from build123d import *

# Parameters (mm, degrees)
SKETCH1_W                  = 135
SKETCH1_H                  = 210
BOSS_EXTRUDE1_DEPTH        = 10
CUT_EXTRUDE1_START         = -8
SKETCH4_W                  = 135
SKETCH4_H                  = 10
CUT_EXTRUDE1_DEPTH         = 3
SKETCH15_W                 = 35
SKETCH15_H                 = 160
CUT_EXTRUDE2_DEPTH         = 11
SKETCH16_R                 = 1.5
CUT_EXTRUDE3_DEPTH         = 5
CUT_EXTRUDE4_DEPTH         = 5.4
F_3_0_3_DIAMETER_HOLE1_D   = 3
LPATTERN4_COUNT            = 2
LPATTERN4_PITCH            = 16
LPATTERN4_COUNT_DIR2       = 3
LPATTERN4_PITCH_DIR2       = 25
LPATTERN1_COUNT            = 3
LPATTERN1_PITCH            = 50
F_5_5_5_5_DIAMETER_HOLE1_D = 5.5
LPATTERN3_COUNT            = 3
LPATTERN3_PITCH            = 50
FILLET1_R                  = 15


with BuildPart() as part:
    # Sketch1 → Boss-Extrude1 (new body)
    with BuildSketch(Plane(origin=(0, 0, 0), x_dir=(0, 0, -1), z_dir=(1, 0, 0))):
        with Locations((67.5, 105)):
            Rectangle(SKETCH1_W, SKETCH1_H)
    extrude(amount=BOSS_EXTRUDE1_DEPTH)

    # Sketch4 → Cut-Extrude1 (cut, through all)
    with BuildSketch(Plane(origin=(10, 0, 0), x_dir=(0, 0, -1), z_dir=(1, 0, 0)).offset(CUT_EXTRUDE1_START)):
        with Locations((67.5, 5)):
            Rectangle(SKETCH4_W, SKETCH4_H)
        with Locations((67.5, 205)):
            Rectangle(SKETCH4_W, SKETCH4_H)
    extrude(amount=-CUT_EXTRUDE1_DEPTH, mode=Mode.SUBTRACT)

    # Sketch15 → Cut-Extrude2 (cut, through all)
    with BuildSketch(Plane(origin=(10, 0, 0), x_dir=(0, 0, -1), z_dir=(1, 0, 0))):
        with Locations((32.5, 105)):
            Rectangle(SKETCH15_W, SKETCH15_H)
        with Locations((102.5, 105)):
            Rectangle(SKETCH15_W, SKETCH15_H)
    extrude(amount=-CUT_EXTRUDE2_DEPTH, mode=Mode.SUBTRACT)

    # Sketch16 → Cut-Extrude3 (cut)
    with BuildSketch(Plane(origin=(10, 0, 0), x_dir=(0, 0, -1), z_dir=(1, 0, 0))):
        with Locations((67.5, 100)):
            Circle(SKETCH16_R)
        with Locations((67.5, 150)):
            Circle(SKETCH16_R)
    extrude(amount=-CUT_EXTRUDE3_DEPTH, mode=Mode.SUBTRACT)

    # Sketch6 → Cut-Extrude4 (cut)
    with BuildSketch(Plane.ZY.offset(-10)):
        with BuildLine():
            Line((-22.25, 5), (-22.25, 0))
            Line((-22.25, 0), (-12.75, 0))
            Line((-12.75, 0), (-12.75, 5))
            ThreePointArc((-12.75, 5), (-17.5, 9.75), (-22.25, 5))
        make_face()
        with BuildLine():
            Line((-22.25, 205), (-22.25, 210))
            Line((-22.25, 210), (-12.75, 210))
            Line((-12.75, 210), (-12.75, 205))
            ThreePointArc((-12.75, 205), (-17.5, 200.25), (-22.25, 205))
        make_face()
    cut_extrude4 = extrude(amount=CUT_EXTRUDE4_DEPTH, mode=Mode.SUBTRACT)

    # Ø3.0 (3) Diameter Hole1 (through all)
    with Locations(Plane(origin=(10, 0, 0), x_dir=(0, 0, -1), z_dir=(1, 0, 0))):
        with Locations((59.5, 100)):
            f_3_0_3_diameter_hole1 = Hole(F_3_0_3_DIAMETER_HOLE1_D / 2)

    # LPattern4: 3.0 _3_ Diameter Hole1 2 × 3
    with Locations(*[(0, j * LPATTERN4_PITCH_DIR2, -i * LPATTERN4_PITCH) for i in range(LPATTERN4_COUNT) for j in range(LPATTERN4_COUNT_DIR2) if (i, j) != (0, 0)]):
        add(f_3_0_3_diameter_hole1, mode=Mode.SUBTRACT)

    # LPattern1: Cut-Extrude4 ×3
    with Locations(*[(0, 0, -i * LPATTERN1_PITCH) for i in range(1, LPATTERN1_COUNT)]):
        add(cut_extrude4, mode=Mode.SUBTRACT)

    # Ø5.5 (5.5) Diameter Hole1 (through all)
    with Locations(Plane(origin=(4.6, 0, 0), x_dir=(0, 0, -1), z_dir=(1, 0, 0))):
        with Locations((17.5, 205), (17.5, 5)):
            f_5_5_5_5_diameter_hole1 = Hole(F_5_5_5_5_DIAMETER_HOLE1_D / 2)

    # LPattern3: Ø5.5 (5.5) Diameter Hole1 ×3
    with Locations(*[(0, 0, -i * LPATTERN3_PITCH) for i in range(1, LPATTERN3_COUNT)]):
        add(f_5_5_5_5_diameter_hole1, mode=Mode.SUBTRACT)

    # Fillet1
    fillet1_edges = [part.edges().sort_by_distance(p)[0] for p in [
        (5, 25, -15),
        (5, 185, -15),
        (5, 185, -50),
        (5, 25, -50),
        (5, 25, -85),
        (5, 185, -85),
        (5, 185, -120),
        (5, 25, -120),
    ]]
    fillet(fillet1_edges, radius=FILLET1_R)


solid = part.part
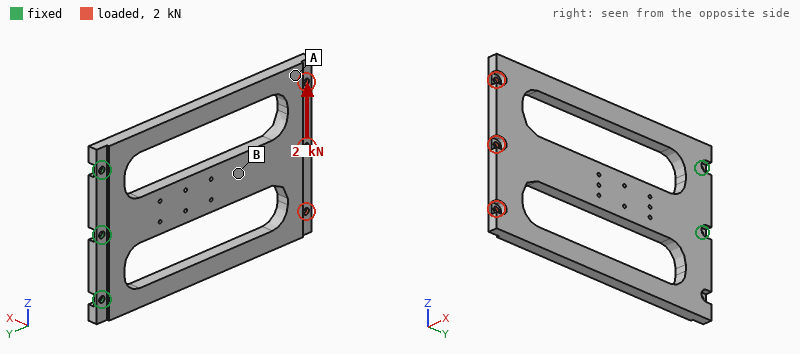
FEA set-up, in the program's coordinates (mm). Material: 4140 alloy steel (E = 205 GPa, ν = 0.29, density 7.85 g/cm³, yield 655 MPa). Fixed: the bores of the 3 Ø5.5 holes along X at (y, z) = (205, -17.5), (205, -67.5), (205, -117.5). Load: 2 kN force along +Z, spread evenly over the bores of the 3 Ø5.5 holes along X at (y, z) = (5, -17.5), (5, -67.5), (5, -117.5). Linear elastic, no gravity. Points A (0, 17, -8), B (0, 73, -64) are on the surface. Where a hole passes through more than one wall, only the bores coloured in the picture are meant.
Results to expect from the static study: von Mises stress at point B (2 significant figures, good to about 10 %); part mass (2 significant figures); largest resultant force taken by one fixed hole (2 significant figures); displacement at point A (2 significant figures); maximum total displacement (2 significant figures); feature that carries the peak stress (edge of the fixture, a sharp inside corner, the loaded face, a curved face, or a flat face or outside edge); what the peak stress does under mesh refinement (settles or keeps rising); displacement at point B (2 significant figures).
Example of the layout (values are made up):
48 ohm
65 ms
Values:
16 MPa
1.3 kg
4.0 kN
0.16 mm
0.16 mm
edge of the fixture
keeps rising
0.11 mm
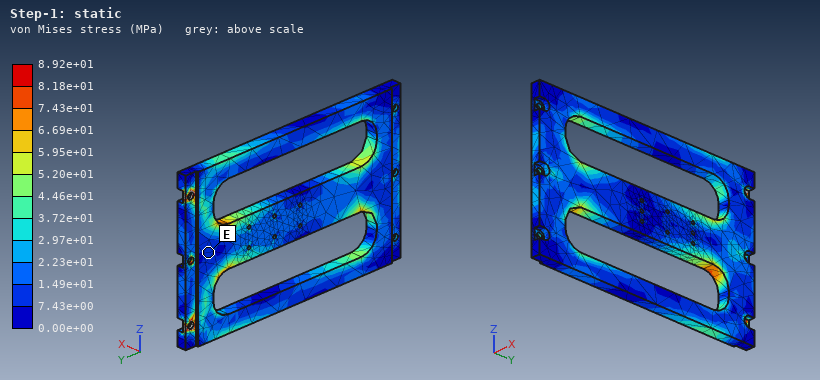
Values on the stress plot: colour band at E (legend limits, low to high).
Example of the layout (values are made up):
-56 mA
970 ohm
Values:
7.43e+00 to 1.49e+01 MPa
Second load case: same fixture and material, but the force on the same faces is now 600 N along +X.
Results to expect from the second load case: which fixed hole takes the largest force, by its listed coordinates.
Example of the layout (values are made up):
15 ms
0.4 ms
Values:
(205, -67.5)
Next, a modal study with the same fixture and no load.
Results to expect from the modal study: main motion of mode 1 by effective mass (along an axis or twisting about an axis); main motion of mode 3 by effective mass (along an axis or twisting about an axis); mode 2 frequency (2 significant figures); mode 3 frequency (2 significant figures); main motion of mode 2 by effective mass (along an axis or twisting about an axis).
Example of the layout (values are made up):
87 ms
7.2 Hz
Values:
along X
along Z
480 Hz
800 Hz
twisting about Y
